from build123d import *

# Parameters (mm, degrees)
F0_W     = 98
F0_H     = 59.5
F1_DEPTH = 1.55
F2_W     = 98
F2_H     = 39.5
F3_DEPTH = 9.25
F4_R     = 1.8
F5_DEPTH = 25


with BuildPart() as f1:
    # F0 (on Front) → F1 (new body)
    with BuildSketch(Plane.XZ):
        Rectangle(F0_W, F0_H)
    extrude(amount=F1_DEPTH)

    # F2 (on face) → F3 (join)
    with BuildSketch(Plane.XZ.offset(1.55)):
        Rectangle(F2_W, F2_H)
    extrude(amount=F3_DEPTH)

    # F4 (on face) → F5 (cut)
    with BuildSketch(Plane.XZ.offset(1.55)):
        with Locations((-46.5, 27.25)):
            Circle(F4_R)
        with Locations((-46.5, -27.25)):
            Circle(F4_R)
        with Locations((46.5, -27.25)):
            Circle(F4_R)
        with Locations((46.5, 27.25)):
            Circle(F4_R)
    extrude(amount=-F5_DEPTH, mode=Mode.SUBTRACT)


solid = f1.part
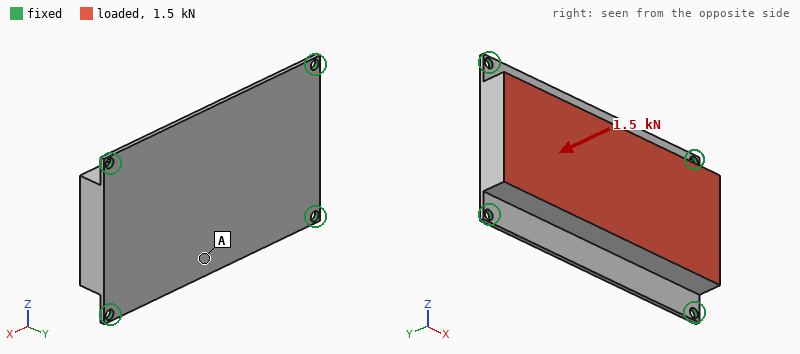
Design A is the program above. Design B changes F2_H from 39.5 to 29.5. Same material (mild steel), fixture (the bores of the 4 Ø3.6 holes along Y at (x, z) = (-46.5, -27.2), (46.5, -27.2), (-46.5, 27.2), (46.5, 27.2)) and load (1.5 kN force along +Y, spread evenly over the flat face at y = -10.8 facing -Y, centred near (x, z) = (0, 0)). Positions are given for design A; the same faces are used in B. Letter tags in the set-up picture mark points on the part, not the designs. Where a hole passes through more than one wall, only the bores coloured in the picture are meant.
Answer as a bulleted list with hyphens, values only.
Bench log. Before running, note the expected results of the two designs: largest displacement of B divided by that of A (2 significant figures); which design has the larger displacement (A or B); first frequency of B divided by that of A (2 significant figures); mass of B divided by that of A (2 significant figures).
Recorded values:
- 2.6
- B
- 0.66
- 0.80
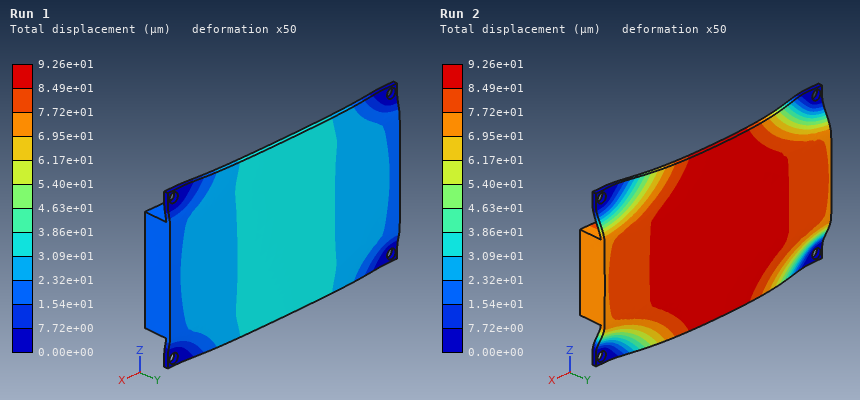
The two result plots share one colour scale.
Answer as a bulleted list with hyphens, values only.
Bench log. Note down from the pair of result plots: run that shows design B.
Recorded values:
- Run 2
